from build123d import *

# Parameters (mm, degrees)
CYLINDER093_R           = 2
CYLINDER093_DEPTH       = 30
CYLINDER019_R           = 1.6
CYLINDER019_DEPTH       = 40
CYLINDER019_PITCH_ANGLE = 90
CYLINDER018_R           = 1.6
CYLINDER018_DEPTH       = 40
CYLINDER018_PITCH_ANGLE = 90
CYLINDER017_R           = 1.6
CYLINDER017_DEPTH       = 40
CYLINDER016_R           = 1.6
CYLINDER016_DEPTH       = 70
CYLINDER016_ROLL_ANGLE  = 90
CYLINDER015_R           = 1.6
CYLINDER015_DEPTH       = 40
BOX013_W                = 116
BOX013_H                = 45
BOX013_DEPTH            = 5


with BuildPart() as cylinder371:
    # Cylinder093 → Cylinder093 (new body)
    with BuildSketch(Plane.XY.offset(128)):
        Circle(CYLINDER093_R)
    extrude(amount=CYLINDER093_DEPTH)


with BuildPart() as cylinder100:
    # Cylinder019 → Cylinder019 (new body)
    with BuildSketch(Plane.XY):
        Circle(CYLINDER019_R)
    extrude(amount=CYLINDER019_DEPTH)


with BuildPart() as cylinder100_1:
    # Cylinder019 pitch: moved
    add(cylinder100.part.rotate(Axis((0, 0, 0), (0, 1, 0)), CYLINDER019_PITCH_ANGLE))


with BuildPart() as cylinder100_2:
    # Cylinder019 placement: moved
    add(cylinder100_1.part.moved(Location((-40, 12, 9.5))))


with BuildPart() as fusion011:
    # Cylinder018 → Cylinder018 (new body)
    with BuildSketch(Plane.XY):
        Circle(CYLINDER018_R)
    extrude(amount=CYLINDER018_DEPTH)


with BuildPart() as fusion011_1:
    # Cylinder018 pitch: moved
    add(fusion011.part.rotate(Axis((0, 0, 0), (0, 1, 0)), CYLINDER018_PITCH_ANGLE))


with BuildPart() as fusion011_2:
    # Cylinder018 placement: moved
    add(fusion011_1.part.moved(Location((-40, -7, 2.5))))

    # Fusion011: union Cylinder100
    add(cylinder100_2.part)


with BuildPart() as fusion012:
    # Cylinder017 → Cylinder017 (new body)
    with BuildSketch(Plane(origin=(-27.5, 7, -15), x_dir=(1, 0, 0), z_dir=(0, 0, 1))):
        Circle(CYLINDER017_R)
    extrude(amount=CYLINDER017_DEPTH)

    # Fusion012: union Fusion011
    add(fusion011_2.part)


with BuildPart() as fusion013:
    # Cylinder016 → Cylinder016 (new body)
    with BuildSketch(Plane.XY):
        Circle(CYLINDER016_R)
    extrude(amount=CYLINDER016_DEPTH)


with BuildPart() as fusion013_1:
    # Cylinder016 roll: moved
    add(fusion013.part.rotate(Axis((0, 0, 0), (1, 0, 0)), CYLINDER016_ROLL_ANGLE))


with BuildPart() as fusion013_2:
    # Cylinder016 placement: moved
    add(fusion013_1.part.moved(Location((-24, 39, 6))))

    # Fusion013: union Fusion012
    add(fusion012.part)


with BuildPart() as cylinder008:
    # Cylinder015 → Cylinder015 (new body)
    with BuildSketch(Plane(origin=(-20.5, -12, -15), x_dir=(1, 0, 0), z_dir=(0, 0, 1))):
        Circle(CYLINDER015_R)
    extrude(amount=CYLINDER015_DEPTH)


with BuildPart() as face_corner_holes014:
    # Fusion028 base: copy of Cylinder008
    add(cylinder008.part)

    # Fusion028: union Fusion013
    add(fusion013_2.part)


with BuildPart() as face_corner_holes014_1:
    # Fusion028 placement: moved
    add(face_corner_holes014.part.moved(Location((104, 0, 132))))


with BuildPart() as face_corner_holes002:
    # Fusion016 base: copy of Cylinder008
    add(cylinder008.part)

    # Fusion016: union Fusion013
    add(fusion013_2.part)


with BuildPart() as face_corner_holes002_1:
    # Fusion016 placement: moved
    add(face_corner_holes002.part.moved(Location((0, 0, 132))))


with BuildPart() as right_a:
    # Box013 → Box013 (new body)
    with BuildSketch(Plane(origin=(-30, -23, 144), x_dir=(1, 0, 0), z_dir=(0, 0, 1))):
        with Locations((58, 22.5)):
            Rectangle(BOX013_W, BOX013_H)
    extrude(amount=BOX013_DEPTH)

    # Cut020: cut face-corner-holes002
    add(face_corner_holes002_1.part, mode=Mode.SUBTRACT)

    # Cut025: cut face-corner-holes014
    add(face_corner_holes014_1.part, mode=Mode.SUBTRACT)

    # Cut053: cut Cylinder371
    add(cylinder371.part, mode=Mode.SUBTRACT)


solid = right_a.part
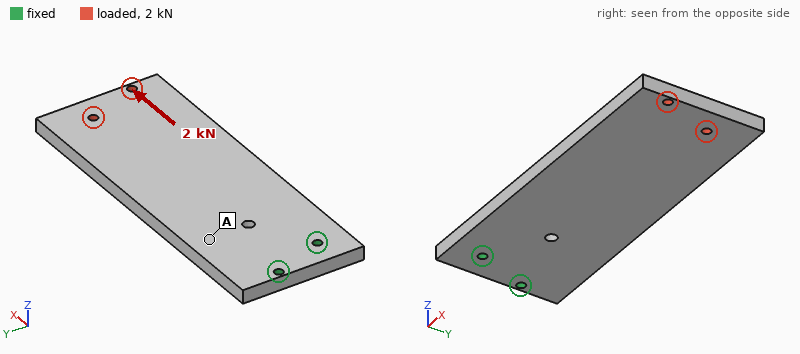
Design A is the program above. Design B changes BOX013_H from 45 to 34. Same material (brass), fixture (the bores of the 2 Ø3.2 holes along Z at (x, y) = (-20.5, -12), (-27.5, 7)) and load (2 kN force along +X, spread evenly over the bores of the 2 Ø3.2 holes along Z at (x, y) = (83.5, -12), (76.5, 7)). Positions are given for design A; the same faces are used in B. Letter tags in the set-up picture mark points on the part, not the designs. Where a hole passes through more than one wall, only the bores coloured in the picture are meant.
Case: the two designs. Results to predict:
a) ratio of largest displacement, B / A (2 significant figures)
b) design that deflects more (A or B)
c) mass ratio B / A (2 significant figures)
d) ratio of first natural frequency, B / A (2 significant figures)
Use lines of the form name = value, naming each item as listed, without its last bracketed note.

ratio of largest displacement, B / A = 1.4
design that deflects more = B
mass ratio B / A = 0.75
ratio of first natural frequency, B / A = 1.0
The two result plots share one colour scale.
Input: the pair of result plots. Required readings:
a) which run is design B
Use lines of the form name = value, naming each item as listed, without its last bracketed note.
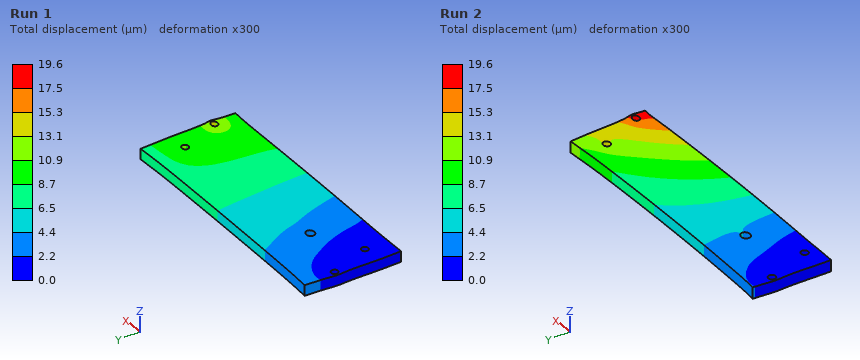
which run is design B = Run 2
